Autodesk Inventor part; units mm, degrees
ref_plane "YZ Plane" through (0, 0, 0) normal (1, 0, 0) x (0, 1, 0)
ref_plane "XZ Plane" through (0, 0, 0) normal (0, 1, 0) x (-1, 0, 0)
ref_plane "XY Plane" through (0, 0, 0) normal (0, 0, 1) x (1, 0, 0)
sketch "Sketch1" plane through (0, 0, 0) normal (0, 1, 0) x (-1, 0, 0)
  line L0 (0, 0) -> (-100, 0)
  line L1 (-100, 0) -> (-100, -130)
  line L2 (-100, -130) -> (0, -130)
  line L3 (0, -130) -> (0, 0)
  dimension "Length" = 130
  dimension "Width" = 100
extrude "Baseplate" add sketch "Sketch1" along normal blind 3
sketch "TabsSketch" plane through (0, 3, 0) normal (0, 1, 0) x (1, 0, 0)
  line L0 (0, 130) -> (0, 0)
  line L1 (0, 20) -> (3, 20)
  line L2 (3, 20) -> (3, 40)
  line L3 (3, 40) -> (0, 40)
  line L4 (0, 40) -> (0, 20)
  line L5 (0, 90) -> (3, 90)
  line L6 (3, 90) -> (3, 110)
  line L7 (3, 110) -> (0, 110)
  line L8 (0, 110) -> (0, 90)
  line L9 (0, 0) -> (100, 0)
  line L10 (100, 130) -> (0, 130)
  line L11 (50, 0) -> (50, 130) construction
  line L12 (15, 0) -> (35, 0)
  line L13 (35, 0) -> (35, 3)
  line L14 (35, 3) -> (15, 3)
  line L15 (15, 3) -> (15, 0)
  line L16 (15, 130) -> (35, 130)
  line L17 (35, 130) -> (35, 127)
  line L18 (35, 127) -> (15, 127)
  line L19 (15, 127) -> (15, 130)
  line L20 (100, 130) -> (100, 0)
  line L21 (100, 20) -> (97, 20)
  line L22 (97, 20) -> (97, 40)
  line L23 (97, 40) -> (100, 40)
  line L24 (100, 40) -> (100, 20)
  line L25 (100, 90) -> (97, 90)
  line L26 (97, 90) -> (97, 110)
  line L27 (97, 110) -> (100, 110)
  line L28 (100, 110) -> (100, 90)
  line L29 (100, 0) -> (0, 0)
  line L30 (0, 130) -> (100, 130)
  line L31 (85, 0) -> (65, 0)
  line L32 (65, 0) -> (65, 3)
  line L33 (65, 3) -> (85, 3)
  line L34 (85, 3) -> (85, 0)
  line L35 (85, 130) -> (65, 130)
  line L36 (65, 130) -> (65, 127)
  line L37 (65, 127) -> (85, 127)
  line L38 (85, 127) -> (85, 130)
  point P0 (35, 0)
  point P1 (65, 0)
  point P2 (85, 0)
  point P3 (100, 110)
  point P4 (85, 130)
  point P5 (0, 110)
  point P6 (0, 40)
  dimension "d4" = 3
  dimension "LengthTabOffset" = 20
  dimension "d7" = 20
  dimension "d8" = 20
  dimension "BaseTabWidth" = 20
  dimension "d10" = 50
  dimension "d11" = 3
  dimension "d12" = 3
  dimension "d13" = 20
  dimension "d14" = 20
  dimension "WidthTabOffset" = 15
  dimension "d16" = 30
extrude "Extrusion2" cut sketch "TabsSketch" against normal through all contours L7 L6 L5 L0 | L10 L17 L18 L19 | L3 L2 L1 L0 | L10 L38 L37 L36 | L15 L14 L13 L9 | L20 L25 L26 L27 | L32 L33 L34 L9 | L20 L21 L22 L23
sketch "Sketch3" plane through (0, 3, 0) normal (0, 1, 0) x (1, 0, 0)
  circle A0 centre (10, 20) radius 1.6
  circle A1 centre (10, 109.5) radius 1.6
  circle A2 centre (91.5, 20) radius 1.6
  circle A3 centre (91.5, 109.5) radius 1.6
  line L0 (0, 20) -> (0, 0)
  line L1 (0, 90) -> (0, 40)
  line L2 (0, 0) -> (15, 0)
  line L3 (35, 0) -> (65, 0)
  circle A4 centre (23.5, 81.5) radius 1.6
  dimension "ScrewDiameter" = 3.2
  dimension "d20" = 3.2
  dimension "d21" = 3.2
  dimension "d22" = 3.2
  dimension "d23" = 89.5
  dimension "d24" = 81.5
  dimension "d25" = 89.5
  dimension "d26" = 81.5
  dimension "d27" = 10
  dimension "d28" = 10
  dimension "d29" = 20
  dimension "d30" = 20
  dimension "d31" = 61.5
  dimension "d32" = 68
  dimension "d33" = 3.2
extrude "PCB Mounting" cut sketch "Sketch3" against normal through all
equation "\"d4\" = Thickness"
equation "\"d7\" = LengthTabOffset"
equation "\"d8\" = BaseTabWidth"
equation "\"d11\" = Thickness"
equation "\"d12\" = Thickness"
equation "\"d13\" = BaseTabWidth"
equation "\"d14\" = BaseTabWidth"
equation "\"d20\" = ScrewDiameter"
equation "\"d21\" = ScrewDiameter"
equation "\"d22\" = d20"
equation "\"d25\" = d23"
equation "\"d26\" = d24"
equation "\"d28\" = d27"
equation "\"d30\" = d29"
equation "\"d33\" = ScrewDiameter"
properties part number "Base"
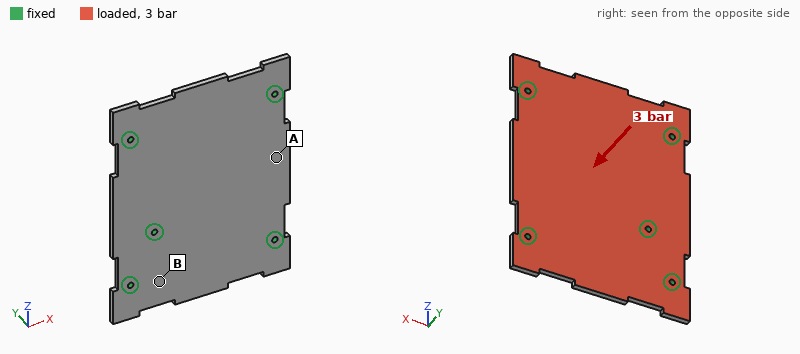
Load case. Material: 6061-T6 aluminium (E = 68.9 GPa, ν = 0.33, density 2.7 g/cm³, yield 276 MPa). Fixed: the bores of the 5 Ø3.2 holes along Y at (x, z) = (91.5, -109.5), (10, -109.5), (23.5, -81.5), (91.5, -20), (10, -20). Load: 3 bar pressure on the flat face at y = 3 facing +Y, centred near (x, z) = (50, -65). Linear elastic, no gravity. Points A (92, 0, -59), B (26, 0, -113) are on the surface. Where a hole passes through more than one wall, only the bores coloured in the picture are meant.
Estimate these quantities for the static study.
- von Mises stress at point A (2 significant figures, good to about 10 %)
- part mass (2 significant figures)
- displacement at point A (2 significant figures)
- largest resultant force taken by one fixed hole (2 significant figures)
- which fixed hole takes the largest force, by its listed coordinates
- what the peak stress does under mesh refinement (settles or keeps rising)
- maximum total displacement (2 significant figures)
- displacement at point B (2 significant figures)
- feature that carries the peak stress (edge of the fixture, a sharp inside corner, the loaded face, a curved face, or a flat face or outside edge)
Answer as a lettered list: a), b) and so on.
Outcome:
a) 69 MPa
b) 100 g
c) 0.37 mm
d) 1.1 kN
e) (23.5, -81.5)
f) keeps rising
g) 0.41 mm
h) 0.097 mm
i) edge of the fixture
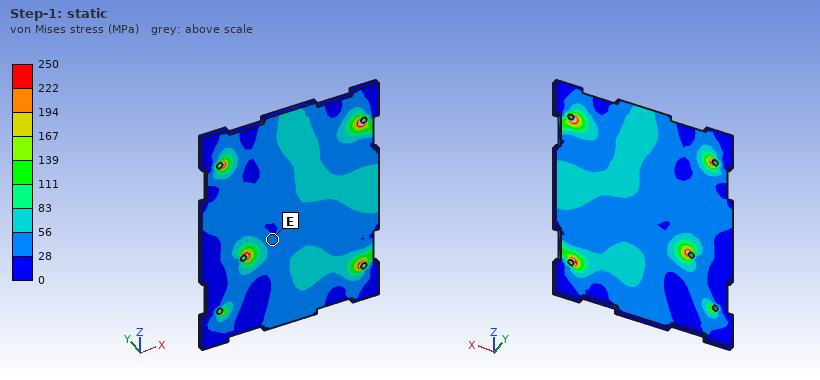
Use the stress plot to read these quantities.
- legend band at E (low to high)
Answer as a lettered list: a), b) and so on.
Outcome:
a) 28 to 56 MPa
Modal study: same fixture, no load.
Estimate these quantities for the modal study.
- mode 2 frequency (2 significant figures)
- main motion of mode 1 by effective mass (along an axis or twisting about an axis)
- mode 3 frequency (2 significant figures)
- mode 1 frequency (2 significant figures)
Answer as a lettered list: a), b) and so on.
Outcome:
a) 2100 Hz
b) along Y
c) 2200 Hz
d) 1700 Hz
